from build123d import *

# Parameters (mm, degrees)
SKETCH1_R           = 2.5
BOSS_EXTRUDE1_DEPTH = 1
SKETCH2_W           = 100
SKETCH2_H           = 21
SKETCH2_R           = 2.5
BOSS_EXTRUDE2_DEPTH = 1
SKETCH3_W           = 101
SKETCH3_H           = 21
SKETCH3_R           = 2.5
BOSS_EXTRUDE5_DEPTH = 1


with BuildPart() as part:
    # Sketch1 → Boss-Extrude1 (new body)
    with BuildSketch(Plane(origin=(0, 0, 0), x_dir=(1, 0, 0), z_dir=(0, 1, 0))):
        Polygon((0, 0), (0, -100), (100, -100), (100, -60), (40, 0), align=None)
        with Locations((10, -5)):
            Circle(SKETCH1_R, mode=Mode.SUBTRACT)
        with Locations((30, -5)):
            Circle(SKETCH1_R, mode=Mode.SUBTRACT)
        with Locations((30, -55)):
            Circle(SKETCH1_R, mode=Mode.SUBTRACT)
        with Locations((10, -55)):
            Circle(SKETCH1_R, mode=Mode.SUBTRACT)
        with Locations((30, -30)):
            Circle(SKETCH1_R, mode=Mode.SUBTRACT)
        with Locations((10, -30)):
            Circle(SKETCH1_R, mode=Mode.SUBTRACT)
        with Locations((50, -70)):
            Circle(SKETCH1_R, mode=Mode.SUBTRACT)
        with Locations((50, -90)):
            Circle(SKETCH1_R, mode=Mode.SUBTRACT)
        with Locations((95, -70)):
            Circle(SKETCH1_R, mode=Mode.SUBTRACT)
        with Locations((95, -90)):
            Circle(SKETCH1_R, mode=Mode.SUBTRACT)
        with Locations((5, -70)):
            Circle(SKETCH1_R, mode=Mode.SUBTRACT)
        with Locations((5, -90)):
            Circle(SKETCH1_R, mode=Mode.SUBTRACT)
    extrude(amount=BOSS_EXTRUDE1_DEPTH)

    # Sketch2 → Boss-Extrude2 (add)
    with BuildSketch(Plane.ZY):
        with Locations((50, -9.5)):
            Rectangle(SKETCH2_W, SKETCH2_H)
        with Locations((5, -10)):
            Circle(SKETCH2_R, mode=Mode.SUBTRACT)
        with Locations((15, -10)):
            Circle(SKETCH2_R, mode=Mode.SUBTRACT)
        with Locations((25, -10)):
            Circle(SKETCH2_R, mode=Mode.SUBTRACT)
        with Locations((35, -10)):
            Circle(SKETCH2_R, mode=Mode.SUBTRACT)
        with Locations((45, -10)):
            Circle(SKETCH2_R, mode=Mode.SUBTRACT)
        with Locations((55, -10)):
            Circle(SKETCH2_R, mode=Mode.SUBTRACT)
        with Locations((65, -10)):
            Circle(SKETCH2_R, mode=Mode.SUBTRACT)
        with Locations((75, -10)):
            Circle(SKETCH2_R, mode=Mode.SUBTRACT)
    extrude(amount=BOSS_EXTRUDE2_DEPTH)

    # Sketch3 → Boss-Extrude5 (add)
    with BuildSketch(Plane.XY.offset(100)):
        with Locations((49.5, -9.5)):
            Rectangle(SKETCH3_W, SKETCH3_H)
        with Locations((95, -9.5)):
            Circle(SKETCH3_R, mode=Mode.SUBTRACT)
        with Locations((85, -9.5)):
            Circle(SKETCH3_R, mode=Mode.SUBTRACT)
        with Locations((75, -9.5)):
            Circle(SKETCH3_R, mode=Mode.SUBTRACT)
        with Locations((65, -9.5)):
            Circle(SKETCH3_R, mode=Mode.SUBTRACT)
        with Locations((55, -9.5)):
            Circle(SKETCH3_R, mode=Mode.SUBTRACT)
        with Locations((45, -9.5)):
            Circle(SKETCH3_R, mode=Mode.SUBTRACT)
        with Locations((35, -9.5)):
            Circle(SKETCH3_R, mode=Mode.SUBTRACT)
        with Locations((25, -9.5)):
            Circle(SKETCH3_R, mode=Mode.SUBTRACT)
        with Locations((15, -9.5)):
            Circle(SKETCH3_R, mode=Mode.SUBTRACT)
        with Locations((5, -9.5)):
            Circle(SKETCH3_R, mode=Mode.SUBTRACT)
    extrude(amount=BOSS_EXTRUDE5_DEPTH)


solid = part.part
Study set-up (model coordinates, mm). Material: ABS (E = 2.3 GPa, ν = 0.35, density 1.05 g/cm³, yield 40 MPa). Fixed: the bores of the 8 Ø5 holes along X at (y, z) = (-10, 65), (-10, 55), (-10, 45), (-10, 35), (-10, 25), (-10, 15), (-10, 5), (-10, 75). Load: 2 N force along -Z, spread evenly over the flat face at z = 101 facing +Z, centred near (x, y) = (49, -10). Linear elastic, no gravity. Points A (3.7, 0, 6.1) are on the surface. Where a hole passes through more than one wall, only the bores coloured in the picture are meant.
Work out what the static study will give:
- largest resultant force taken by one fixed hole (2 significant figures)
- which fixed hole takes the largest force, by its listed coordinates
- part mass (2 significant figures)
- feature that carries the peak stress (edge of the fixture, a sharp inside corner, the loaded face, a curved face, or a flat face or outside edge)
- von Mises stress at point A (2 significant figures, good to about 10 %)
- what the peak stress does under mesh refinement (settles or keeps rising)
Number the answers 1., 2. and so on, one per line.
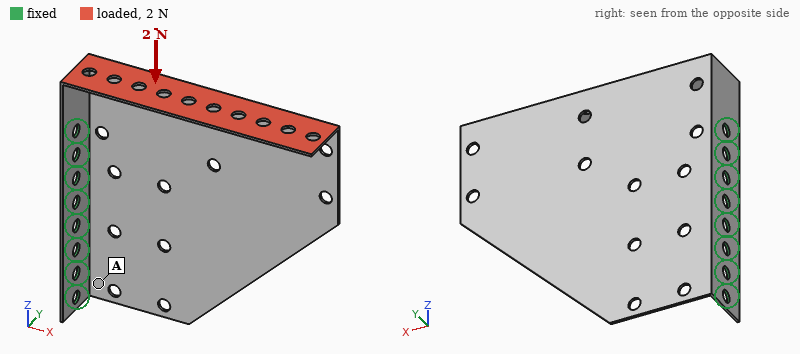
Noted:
1. 1.1 N
2. (-10, 75)
3. 12 g
4. edge of the fixture
5. 0.41 MPa
6. keeps rising
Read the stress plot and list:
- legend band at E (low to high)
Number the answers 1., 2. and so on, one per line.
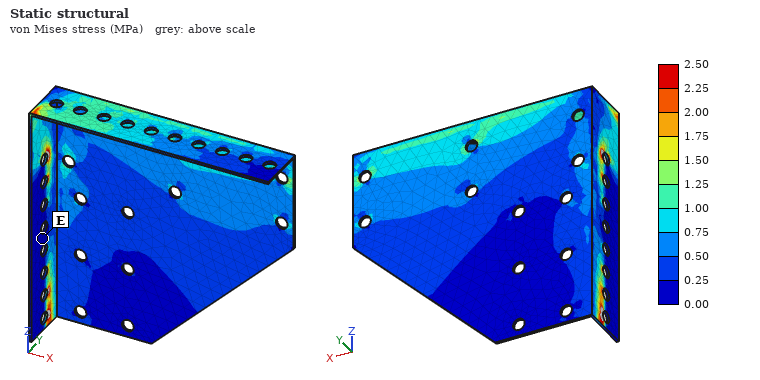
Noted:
1. 0.00 to 0.25 MPa
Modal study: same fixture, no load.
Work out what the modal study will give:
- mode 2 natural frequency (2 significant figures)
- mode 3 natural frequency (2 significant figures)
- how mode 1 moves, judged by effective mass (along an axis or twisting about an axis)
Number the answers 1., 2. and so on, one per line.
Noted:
1. 75 Hz
2. 170 Hz
3. along Y
